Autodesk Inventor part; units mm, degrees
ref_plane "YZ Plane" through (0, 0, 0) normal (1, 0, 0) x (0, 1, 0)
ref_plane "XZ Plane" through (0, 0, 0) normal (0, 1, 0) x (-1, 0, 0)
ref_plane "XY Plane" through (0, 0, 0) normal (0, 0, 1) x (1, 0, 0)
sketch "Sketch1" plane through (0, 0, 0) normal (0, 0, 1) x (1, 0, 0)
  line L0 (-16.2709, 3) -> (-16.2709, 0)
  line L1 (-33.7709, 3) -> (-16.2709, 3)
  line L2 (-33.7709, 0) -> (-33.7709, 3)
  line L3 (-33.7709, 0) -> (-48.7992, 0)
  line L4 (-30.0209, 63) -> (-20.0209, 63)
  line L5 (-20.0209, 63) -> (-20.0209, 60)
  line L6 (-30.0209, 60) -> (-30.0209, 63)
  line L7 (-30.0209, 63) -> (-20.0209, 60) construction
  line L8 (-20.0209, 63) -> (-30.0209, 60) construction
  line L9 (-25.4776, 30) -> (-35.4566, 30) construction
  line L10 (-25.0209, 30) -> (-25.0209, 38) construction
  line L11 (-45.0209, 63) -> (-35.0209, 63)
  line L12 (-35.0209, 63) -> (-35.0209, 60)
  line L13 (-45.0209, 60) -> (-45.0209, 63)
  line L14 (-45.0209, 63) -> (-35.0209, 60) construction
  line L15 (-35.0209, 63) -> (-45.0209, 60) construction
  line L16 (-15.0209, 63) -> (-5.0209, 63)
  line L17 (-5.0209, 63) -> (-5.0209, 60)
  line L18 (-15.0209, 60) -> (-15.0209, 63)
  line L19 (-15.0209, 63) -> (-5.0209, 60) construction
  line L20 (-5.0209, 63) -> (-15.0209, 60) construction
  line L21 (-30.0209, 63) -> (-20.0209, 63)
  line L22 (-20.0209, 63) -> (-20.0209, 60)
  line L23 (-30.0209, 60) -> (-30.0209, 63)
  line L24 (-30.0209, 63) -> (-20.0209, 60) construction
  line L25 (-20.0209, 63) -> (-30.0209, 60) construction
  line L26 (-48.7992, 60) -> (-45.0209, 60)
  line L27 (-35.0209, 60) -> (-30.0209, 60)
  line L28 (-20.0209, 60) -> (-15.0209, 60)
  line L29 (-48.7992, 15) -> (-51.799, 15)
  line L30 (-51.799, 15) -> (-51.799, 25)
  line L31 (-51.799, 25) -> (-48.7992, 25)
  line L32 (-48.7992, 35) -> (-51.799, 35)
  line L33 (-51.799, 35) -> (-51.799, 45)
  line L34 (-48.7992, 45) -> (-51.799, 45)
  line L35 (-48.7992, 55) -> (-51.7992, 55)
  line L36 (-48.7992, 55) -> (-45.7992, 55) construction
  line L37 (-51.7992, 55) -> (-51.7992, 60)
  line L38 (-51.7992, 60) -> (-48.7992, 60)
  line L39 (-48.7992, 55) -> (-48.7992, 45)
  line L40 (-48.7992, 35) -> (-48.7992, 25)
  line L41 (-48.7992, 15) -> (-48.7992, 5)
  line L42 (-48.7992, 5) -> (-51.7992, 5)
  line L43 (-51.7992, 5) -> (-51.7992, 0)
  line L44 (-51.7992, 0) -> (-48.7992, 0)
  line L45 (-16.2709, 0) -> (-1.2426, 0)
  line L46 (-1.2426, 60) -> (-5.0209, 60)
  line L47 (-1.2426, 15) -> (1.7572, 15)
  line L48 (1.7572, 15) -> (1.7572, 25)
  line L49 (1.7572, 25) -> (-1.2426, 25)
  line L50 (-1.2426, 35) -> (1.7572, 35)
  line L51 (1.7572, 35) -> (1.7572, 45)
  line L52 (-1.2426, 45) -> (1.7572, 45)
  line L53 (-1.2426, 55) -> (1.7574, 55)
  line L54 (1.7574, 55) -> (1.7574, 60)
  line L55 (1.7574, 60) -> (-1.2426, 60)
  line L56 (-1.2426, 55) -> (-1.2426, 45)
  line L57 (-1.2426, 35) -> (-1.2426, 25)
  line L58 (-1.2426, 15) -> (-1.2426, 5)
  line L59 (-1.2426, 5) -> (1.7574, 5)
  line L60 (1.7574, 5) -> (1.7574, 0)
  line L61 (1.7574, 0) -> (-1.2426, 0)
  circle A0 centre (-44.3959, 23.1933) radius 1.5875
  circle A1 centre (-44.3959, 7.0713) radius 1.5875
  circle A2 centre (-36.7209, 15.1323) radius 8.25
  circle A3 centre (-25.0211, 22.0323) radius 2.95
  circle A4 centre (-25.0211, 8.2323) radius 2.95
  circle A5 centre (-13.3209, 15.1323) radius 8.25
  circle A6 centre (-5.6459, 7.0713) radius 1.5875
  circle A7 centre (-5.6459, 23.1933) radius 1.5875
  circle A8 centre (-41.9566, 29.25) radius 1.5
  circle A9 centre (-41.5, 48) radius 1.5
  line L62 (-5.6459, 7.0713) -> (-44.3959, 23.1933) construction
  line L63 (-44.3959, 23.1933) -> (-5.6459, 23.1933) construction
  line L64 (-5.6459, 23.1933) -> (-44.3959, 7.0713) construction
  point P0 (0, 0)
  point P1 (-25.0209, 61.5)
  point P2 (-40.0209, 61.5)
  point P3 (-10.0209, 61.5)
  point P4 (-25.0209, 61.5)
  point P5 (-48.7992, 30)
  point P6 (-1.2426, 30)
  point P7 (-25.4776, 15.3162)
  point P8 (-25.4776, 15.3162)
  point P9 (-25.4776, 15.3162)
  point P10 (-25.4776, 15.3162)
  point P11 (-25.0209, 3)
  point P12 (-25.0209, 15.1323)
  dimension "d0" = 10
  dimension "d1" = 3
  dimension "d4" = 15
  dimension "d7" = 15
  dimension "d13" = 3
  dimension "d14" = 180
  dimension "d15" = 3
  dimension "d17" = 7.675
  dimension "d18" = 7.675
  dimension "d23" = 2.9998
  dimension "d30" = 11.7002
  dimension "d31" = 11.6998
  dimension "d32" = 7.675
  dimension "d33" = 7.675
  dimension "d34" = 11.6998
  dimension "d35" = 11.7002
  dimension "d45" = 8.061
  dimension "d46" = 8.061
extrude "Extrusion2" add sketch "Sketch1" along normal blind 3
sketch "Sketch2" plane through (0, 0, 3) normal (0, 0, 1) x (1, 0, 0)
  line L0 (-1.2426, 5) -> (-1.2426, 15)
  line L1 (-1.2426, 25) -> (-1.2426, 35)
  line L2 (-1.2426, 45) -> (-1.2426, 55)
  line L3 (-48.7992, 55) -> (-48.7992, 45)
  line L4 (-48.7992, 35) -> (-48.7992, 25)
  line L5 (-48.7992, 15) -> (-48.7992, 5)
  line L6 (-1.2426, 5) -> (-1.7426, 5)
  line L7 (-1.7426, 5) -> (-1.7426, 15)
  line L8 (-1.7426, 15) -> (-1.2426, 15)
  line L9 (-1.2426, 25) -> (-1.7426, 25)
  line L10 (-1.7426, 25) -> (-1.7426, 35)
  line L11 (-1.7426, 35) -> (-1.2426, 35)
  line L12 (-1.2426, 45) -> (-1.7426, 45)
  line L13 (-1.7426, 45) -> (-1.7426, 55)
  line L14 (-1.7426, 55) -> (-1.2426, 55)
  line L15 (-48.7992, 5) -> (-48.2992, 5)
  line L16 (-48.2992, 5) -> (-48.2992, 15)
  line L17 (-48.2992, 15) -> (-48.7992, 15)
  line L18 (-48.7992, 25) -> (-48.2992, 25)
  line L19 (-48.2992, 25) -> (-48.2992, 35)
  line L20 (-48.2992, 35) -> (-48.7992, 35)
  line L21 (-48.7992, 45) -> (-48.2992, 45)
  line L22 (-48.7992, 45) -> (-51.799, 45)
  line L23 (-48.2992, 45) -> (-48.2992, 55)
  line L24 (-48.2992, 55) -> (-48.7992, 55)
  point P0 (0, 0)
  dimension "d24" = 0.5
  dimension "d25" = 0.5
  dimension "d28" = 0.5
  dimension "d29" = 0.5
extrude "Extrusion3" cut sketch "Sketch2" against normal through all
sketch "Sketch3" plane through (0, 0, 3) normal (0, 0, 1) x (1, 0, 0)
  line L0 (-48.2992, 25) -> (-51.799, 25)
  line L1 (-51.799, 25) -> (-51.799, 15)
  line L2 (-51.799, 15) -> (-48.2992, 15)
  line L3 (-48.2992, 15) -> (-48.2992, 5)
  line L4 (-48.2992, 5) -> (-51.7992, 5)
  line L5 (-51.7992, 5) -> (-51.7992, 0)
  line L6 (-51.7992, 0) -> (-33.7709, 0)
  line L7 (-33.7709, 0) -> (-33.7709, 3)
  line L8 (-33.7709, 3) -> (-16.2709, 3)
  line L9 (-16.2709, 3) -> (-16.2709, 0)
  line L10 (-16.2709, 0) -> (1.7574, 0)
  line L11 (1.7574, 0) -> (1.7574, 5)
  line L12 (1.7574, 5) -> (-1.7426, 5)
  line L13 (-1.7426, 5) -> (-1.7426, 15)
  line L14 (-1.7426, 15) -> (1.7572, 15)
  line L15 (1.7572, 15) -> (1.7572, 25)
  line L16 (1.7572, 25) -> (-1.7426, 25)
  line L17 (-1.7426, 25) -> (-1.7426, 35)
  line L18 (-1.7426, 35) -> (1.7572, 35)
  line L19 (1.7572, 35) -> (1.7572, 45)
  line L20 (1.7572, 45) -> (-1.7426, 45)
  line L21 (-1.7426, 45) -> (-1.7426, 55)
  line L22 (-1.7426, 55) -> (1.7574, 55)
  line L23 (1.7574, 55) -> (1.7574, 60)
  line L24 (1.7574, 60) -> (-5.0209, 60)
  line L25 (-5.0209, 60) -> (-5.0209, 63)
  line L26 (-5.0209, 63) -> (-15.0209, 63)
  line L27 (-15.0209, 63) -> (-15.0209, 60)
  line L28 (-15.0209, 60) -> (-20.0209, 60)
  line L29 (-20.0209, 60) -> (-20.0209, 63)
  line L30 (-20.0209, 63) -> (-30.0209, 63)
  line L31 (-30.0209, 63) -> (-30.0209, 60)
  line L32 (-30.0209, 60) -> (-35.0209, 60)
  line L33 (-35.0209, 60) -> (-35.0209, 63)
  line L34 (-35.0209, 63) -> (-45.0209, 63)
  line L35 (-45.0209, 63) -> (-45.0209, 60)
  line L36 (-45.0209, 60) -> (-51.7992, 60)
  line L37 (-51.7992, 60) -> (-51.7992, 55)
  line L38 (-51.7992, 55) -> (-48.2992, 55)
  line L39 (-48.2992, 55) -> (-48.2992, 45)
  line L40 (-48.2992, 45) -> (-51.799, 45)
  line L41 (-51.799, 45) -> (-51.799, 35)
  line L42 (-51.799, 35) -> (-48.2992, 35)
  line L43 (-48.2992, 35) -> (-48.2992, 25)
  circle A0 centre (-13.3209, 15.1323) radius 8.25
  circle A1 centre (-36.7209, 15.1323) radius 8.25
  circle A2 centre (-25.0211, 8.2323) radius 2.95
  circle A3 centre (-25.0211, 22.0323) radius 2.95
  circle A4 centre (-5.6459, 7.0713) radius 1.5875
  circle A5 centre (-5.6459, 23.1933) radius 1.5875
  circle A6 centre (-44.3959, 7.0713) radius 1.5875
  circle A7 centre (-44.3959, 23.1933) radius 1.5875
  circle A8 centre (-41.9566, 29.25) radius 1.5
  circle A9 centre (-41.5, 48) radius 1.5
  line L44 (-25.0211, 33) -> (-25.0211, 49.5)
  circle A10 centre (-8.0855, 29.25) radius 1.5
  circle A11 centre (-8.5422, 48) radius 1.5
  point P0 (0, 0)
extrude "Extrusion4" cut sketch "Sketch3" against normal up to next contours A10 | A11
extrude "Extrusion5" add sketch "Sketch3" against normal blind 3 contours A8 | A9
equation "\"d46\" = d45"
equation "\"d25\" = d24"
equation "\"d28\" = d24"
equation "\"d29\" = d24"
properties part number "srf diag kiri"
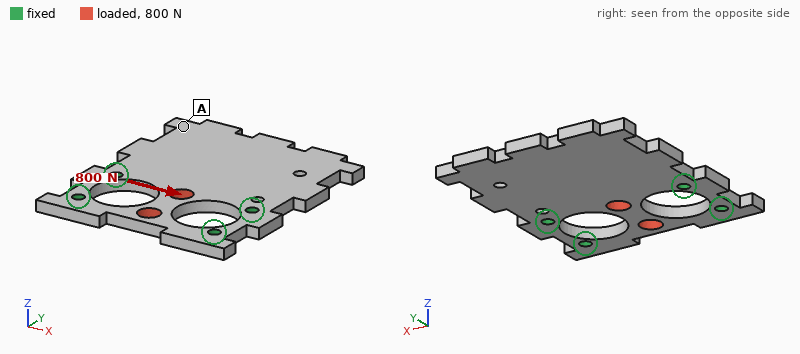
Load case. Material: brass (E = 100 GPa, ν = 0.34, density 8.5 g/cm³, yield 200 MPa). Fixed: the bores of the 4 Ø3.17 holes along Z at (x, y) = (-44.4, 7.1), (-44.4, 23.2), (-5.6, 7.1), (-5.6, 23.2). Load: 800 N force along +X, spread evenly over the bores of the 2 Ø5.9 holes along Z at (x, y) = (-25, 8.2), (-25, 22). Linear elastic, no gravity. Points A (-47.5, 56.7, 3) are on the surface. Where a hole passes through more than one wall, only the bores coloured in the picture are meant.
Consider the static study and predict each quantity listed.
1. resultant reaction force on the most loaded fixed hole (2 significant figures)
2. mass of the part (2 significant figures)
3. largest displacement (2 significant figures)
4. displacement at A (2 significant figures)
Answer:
230 N
64 g
4.9 µm
0.85 µm
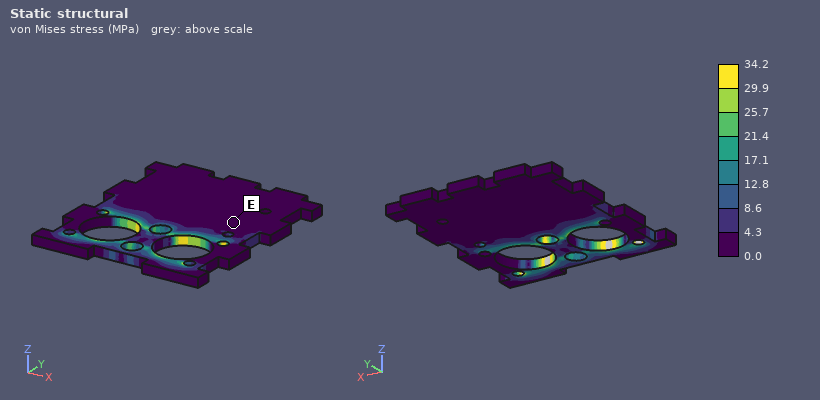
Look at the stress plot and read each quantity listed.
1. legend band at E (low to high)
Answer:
0.0 to 4.3 MPa
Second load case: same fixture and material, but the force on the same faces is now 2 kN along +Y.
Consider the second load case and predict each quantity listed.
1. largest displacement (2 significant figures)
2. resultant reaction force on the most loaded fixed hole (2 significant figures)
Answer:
24 µm
840 N
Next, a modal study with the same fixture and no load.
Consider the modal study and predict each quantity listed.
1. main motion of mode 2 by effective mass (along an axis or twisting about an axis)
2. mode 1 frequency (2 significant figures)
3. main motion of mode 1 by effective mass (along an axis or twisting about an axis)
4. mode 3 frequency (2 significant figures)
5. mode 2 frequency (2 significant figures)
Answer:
twisting about Y
880 Hz
along Z
5000 Hz
2100 Hz
